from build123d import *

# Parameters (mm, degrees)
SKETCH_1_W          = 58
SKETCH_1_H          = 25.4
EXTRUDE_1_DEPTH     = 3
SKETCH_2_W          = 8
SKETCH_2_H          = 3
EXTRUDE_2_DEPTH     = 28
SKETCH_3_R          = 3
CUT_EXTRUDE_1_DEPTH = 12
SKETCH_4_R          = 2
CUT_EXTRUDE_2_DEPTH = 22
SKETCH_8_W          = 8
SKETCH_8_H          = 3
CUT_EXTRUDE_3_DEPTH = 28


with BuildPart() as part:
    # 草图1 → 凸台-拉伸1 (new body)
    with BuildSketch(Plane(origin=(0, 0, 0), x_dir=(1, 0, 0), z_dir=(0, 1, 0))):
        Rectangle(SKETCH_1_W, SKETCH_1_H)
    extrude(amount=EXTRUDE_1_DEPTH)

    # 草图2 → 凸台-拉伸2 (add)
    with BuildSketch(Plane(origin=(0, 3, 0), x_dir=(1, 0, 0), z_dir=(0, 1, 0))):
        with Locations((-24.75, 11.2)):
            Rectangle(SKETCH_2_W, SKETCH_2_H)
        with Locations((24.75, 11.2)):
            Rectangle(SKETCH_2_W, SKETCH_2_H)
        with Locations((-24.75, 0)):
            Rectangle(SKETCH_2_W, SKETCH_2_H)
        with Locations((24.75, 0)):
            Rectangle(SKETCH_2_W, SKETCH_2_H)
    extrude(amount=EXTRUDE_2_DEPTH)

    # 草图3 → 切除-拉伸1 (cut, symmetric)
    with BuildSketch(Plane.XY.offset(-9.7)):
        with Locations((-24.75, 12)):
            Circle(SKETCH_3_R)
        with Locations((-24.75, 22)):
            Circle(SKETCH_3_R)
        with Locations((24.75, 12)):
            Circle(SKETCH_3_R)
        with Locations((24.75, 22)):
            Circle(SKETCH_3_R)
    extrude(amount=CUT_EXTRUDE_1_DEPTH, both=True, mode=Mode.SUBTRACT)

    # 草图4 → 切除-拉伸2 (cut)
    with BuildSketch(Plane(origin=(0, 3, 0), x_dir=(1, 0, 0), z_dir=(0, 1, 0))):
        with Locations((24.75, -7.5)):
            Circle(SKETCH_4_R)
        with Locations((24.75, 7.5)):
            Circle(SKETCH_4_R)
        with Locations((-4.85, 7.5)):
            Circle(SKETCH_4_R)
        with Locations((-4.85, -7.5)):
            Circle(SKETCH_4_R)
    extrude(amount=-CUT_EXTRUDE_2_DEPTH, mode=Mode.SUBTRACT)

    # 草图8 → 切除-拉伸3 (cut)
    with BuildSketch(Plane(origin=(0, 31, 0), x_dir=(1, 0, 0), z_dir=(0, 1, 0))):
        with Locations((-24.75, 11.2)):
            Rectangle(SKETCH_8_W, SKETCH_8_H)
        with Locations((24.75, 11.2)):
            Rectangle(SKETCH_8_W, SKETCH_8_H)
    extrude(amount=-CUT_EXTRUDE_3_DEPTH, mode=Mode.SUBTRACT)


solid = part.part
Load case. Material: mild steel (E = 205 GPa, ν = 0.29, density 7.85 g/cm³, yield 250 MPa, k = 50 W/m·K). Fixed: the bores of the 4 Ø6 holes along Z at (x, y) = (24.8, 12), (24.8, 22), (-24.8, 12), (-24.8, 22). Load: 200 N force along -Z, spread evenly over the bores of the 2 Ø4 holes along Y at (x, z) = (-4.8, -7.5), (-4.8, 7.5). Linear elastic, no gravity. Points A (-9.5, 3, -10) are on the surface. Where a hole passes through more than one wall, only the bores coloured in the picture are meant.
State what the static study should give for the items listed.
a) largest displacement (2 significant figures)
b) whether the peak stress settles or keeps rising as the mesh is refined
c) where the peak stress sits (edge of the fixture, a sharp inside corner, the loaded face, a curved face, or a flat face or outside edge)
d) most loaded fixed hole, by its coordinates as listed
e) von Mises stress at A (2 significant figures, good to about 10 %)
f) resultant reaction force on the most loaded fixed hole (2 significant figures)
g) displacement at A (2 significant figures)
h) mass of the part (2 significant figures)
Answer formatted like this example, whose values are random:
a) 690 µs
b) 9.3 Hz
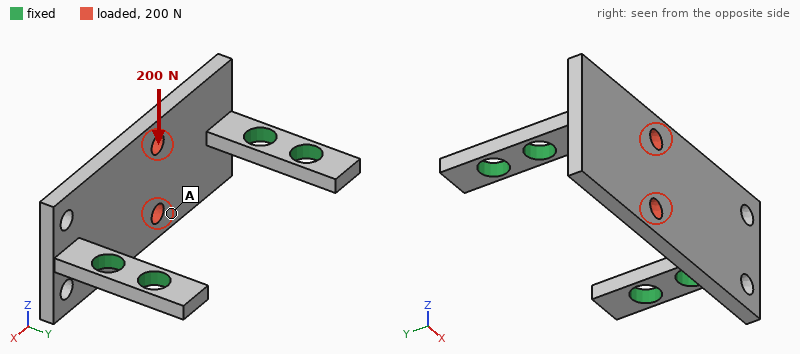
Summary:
a) 14 µm
b) keeps rising
c) edge of the fixture
d) (-24.8, 12)
e) 6.2 MPa
f) 120 N
g) 10 µm
h) 41 g
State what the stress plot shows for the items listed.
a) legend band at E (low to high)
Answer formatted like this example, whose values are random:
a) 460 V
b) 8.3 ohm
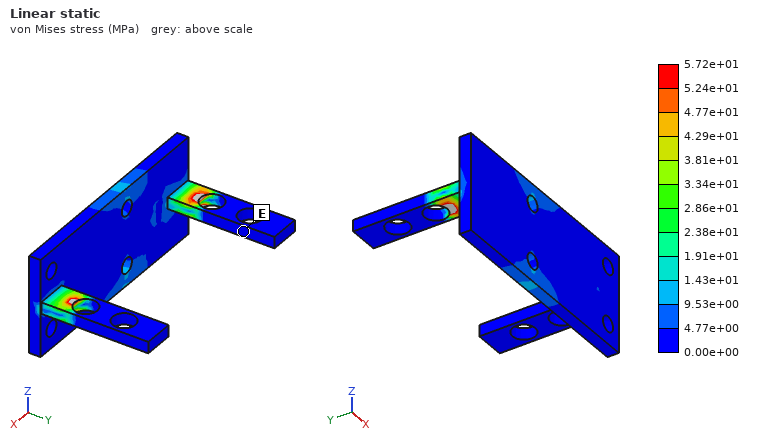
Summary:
a) 0.00e+00 to 4.77e+00 MPa
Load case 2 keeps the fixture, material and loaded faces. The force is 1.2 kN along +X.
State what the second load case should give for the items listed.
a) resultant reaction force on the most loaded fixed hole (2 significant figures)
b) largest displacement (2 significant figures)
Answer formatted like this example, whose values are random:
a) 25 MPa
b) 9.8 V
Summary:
a) 620 N
b) 9.0 µm
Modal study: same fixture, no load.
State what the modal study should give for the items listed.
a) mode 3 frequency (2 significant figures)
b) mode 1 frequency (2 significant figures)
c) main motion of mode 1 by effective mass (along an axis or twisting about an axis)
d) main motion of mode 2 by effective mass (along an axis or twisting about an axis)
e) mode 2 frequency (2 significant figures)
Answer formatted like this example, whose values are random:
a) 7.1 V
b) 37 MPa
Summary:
a) 6800 Hz
b) 3000 Hz
c) along Z
d) along Y
e) 5600 Hz
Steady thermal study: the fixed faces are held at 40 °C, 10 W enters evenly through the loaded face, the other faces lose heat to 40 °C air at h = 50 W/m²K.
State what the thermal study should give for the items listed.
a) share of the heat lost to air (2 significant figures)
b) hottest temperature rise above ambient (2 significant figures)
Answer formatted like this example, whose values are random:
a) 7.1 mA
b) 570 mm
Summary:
a) 46 %
b) 44 K
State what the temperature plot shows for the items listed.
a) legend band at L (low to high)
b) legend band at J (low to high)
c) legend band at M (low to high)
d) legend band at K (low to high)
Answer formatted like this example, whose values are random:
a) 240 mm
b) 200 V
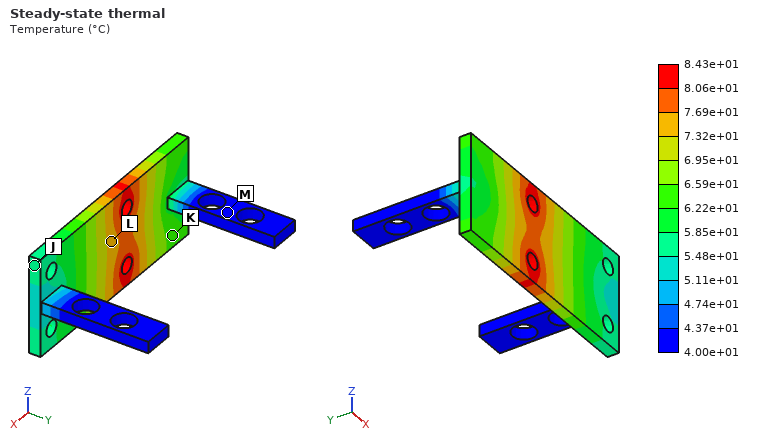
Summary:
a) 7.32e+01 to 7.69e+01 °C
b) 5.48e+01 to 5.85e+01 °C
c) 4.00e+01 to 4.37e+01 °C
d) 6.22e+01 to 6.59e+01 °C
